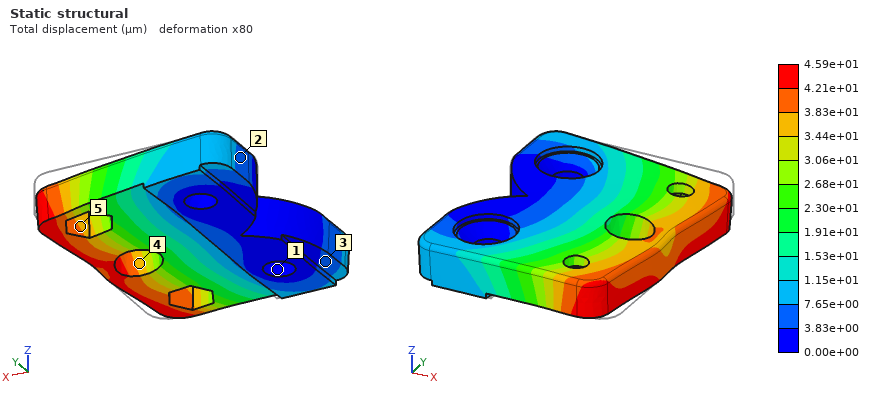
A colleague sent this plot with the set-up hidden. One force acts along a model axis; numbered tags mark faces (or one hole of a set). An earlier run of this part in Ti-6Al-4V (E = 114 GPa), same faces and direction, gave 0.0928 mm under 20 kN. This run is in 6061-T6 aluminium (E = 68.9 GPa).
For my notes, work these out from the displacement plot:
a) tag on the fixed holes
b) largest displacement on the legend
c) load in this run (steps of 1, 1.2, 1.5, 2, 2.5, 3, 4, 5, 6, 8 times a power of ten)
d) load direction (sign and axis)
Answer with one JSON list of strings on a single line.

["1", "4.59e+01 µm", "6 kN", "-Y"]
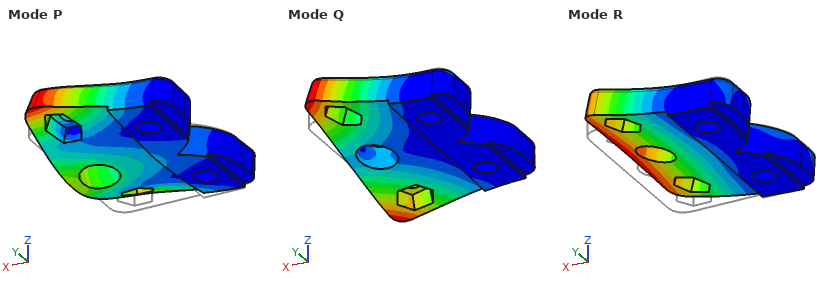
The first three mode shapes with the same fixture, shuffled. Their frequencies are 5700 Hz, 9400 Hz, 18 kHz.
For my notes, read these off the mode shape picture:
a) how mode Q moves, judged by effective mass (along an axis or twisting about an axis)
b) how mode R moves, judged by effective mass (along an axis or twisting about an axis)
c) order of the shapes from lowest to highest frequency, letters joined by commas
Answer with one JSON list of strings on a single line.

["twisting about X", "along Z", "R, Q, P"]
